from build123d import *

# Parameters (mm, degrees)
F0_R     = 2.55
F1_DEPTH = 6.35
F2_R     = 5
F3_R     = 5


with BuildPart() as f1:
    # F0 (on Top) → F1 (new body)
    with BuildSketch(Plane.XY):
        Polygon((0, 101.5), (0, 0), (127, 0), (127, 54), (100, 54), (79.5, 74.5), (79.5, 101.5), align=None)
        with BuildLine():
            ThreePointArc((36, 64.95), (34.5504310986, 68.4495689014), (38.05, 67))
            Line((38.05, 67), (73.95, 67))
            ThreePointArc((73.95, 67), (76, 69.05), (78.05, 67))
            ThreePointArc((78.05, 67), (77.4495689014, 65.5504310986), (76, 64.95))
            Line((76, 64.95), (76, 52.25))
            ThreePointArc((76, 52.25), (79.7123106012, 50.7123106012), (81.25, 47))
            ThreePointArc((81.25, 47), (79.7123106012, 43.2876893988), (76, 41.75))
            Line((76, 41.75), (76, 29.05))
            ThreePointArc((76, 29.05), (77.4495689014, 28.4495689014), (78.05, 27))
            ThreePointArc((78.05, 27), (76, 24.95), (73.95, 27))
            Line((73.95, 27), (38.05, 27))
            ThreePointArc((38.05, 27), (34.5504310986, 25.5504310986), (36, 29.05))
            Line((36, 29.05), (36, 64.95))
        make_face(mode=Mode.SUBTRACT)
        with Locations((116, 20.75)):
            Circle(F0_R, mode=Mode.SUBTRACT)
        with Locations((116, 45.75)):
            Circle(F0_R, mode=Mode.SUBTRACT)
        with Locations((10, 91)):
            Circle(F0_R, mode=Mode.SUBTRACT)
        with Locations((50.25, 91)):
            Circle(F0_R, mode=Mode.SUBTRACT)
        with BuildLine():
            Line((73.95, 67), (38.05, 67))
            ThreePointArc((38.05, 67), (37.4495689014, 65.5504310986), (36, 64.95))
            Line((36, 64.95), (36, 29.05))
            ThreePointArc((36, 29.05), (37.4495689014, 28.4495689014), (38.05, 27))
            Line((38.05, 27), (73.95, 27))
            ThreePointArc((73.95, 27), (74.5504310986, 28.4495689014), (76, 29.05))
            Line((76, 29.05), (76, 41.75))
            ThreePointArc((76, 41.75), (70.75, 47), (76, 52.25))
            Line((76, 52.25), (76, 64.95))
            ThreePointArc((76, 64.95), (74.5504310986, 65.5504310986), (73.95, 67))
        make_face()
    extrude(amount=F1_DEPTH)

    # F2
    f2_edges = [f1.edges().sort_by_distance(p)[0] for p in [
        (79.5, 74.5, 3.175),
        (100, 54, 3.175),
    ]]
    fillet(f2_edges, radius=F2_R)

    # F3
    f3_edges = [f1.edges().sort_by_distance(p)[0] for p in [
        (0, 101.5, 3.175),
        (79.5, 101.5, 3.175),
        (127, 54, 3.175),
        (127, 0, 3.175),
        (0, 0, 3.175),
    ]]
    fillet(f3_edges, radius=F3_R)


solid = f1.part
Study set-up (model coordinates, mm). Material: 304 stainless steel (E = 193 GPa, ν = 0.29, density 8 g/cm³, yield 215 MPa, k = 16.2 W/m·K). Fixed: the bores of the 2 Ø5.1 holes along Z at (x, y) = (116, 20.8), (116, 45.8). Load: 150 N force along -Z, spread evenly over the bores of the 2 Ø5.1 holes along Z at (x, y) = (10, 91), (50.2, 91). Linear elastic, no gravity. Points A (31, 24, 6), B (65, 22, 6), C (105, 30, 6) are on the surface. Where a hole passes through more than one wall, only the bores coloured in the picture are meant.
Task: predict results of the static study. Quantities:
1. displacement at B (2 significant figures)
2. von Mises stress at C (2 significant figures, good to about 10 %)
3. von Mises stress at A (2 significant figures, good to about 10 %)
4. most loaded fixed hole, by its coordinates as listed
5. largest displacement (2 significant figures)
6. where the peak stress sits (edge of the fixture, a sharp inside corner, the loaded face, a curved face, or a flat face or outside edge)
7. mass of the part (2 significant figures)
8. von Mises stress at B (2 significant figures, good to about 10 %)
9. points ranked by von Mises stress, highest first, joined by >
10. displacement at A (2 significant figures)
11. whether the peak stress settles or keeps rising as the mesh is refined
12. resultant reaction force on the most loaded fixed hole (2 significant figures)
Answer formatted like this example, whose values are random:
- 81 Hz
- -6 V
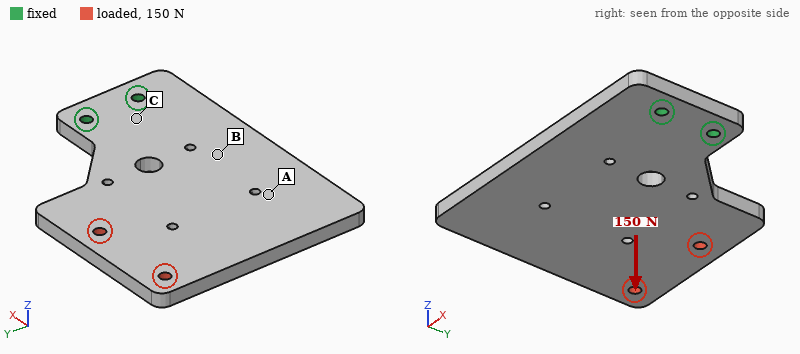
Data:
- 0.051 mm
- 31 MPa
- 9.1 MPa
- (116, 45.8)
- 0.33 mm
- edge of the fixture
- 540 g
- 20 MPa
- C > B > A
- 0.12 mm
- keeps rising
- 320 N
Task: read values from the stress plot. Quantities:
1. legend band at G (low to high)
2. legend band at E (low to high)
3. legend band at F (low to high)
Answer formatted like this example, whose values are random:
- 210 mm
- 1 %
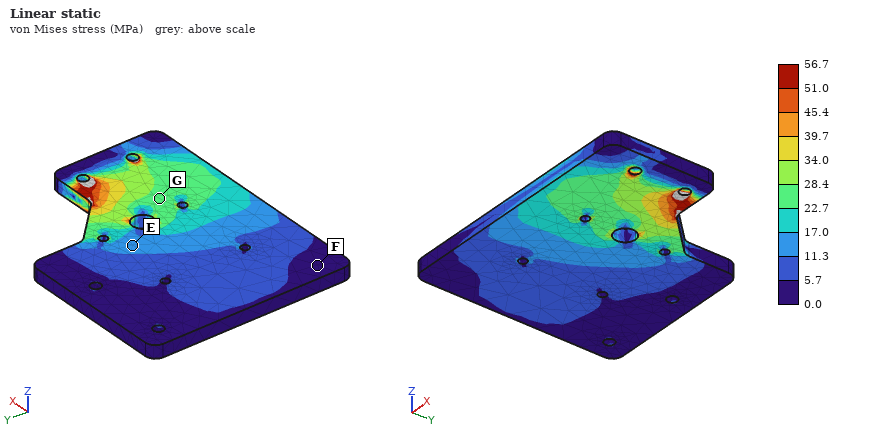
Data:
- 22.7 to 28.4 MPa
- 11.3 to 17.0 MPa
- 0.0 to 5.7 MPa
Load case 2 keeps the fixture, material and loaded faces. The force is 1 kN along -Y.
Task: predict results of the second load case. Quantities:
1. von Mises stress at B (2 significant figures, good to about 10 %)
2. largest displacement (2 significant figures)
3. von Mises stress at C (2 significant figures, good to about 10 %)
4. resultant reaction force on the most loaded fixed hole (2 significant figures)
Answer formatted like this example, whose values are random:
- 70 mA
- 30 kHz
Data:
- 7.5 MPa
- 40 µm
- 17 MPa
- 3.1 kN
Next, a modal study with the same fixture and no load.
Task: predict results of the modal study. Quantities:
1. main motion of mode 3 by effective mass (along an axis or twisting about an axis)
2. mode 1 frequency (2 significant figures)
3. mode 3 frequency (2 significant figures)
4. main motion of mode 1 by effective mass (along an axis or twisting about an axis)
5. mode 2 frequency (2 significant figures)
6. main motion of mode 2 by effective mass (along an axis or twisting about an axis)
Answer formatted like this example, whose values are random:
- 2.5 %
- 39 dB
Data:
- along Y
- 270 Hz
- 1600 Hz
- along Z
- 700 Hz
- twisting about X
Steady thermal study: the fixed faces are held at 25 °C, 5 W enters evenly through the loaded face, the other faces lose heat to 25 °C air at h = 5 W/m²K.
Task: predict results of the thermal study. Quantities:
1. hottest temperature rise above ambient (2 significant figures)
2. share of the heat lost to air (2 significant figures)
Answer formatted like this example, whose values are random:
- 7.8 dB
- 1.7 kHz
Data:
- 56 K
- 58 %
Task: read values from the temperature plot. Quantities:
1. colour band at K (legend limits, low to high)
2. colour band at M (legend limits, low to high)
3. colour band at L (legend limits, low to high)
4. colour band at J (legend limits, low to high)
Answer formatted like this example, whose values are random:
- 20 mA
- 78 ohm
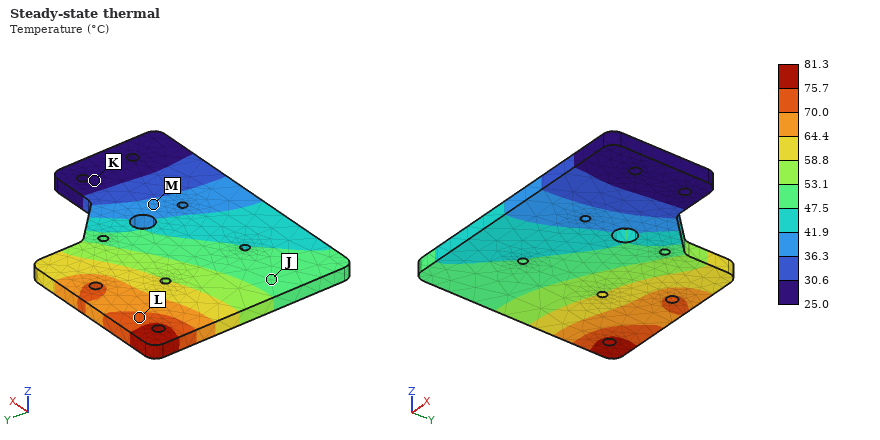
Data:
- 25.0 to 30.6 °C
- 36.3 to 41.9 °C
- 70.0 to 75.7 °C
- 47.5 to 53.1 °C
